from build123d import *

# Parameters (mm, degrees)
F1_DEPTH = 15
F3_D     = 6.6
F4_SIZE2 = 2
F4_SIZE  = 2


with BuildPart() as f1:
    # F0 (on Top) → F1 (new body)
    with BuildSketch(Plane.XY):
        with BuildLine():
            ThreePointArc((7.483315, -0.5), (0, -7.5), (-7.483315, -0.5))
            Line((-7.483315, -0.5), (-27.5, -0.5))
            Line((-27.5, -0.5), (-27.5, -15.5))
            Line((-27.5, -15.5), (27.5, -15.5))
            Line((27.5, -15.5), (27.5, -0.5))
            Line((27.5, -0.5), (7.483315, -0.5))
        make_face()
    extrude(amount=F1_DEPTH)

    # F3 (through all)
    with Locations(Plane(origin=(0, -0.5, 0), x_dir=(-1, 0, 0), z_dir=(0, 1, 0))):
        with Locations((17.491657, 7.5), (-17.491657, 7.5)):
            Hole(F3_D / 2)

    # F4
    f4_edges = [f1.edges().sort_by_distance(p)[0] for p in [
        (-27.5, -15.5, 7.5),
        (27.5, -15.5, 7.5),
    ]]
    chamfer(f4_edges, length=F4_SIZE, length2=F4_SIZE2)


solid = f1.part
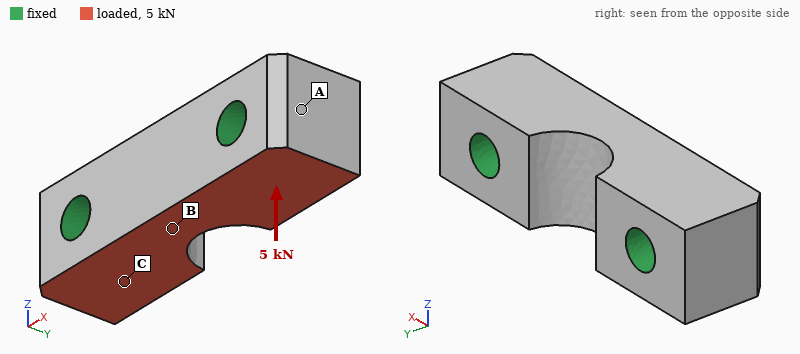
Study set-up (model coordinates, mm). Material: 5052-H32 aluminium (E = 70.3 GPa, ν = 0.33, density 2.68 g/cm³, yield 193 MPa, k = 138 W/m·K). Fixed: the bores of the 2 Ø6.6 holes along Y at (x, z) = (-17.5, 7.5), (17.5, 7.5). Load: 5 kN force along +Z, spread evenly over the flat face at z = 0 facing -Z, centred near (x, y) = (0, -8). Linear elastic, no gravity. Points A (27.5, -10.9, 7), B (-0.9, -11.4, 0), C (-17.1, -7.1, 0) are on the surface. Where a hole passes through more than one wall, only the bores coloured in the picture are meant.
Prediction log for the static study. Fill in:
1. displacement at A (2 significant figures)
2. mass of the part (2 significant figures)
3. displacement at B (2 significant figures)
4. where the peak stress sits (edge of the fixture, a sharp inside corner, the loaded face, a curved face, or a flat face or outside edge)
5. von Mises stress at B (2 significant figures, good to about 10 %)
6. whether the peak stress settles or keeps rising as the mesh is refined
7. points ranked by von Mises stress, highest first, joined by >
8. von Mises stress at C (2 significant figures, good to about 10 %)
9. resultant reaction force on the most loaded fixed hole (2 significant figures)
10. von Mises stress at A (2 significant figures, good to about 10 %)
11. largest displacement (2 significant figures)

0.79 µm
27 g
3.8 µm
edge of the fixture
10 MPa
keeps rising
C > B > A
16 MPa
2.5 kN
4.3 MPa
4.3 µm
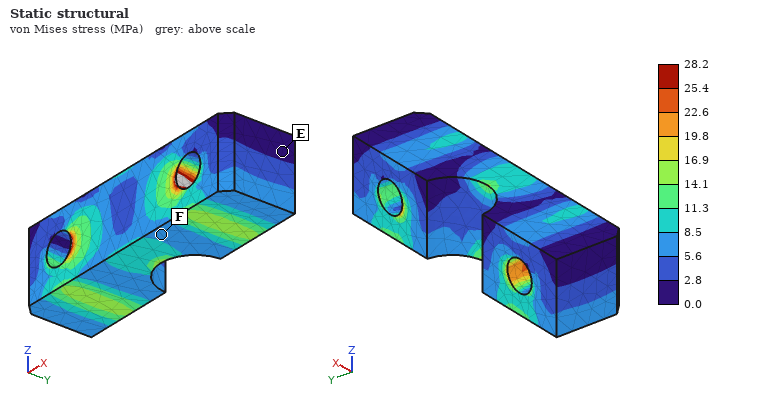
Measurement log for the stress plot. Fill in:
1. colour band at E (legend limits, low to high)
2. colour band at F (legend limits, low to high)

0.0 to 2.8 MPa
5.6 to 8.5 MPa
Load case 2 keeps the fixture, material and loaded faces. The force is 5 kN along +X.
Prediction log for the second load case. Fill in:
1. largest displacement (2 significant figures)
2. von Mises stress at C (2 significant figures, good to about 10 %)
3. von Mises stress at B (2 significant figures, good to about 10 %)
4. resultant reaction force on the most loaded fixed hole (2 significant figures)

4.4 µm
12 MPa
13 MPa
2.6 kN
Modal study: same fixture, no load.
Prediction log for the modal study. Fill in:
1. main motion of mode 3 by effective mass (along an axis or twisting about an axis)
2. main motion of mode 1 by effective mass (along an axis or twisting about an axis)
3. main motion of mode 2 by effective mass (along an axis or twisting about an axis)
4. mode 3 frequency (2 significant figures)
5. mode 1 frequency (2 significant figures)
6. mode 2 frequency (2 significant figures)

twisting about X
along Z
along Y
57 kHz
38 kHz
44 kHz
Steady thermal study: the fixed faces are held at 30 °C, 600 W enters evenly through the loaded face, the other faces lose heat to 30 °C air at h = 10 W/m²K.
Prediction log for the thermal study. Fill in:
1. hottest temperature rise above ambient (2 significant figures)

74 K
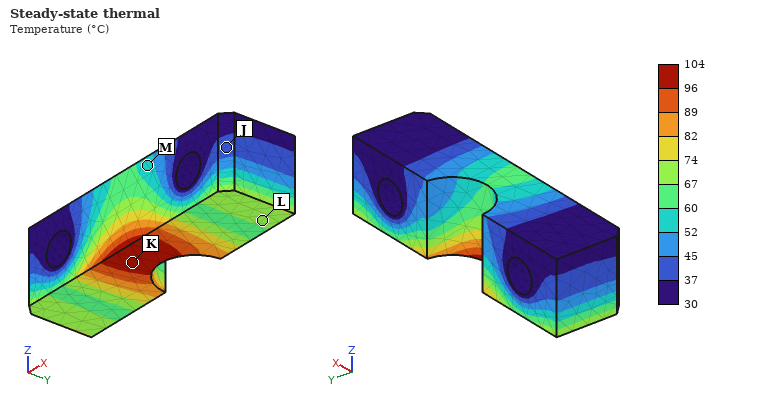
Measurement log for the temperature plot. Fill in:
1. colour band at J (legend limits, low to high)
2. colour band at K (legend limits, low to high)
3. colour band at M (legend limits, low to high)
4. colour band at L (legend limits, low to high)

37 to 45 °C
96 to 104 °C
52 to 60 °C
67 to 74 °C
